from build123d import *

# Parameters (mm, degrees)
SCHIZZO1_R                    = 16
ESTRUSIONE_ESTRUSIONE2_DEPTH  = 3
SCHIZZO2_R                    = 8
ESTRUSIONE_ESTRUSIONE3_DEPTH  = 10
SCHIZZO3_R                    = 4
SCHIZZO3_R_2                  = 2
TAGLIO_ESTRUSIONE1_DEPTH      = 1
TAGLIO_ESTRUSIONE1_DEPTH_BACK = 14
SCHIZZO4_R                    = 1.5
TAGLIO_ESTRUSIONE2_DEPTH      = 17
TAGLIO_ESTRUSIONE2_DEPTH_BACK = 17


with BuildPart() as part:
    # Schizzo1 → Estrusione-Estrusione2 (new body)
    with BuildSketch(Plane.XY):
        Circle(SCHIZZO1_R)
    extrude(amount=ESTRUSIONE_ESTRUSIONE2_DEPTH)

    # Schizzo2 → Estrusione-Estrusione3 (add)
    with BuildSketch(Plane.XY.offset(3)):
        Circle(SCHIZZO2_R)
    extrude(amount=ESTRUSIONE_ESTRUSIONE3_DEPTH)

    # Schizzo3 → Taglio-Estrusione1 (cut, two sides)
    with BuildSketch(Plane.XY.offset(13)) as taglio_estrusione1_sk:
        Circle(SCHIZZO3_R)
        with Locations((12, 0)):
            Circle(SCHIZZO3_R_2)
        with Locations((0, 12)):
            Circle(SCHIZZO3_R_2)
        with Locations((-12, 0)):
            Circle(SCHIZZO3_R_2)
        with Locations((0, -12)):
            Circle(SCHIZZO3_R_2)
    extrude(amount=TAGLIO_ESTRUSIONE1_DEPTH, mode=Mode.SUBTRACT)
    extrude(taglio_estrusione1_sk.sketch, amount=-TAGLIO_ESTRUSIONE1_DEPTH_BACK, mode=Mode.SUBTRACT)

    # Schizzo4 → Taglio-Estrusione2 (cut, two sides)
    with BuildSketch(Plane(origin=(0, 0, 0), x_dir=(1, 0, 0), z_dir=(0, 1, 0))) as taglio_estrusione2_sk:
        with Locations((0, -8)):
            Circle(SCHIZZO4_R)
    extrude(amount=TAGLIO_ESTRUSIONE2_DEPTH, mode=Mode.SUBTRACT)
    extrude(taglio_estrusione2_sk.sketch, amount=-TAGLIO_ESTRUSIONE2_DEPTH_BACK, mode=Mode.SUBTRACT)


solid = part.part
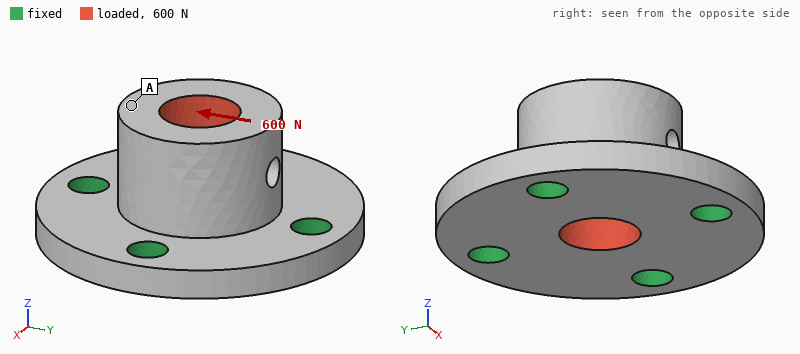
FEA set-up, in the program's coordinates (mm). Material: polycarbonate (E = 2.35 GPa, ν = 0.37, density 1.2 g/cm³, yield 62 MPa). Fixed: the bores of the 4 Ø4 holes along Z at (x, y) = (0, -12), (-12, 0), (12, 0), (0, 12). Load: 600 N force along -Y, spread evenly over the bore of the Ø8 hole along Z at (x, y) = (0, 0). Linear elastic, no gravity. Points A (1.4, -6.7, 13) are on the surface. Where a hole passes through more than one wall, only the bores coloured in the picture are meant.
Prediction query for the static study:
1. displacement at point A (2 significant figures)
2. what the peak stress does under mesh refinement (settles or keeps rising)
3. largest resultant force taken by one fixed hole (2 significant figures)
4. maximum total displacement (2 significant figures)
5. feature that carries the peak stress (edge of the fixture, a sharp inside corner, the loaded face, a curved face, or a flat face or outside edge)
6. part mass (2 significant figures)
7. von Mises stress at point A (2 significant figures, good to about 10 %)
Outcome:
0.11 mm
keeps rising
240 N
0.11 mm
edge of the fixture
4.3 g
3.0 MPa
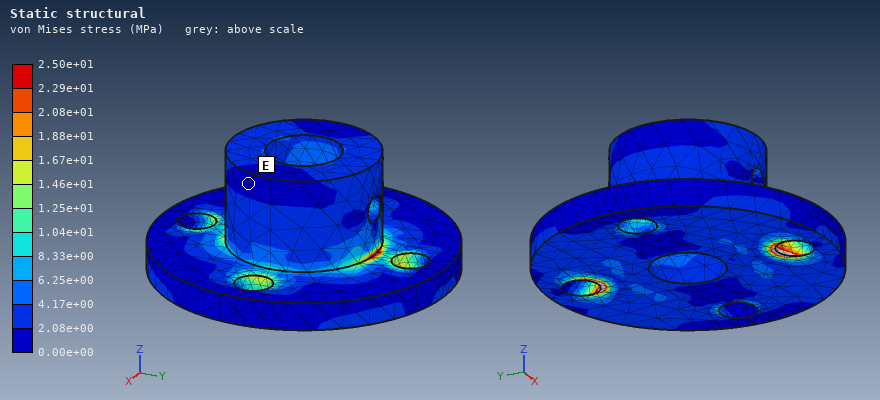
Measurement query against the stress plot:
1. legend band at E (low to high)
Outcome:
0.00e+00 to 2.08e+00 MPa
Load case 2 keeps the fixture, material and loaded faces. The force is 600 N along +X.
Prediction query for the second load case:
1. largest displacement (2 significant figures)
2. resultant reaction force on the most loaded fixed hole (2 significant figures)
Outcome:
0.11 mm
240 N
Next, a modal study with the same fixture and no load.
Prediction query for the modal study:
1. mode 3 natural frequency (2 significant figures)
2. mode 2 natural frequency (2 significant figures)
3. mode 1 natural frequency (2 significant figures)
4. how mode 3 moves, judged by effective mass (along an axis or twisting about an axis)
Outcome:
11 kHz
8700 Hz
8600 Hz
along Z
